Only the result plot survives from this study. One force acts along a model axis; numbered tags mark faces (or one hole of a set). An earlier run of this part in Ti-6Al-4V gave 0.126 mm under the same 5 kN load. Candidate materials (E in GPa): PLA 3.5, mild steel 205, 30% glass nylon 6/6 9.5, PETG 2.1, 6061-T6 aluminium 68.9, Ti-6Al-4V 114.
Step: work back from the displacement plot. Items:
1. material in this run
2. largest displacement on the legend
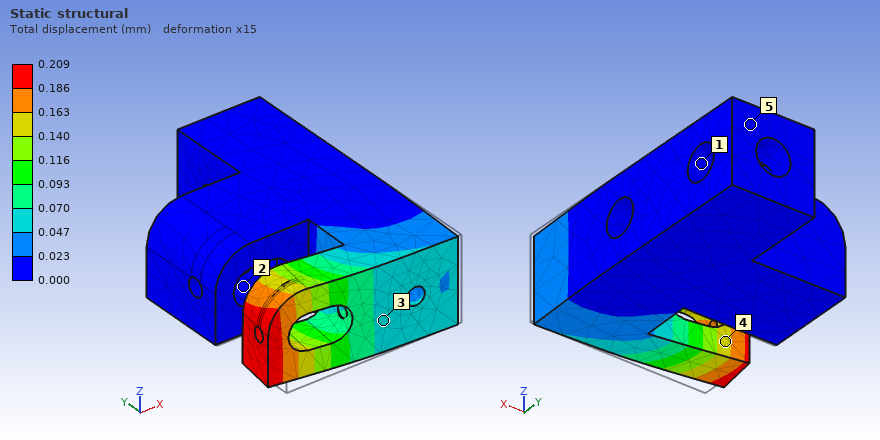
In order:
6061-T6 aluminium
0.209 mm
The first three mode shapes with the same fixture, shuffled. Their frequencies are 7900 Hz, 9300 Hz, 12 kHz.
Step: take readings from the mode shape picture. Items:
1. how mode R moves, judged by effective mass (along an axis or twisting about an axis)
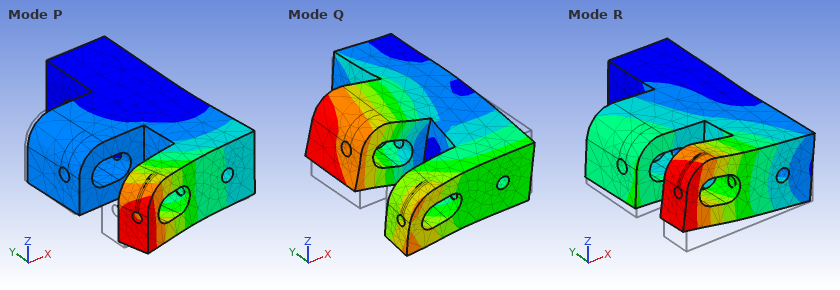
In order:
along Z
